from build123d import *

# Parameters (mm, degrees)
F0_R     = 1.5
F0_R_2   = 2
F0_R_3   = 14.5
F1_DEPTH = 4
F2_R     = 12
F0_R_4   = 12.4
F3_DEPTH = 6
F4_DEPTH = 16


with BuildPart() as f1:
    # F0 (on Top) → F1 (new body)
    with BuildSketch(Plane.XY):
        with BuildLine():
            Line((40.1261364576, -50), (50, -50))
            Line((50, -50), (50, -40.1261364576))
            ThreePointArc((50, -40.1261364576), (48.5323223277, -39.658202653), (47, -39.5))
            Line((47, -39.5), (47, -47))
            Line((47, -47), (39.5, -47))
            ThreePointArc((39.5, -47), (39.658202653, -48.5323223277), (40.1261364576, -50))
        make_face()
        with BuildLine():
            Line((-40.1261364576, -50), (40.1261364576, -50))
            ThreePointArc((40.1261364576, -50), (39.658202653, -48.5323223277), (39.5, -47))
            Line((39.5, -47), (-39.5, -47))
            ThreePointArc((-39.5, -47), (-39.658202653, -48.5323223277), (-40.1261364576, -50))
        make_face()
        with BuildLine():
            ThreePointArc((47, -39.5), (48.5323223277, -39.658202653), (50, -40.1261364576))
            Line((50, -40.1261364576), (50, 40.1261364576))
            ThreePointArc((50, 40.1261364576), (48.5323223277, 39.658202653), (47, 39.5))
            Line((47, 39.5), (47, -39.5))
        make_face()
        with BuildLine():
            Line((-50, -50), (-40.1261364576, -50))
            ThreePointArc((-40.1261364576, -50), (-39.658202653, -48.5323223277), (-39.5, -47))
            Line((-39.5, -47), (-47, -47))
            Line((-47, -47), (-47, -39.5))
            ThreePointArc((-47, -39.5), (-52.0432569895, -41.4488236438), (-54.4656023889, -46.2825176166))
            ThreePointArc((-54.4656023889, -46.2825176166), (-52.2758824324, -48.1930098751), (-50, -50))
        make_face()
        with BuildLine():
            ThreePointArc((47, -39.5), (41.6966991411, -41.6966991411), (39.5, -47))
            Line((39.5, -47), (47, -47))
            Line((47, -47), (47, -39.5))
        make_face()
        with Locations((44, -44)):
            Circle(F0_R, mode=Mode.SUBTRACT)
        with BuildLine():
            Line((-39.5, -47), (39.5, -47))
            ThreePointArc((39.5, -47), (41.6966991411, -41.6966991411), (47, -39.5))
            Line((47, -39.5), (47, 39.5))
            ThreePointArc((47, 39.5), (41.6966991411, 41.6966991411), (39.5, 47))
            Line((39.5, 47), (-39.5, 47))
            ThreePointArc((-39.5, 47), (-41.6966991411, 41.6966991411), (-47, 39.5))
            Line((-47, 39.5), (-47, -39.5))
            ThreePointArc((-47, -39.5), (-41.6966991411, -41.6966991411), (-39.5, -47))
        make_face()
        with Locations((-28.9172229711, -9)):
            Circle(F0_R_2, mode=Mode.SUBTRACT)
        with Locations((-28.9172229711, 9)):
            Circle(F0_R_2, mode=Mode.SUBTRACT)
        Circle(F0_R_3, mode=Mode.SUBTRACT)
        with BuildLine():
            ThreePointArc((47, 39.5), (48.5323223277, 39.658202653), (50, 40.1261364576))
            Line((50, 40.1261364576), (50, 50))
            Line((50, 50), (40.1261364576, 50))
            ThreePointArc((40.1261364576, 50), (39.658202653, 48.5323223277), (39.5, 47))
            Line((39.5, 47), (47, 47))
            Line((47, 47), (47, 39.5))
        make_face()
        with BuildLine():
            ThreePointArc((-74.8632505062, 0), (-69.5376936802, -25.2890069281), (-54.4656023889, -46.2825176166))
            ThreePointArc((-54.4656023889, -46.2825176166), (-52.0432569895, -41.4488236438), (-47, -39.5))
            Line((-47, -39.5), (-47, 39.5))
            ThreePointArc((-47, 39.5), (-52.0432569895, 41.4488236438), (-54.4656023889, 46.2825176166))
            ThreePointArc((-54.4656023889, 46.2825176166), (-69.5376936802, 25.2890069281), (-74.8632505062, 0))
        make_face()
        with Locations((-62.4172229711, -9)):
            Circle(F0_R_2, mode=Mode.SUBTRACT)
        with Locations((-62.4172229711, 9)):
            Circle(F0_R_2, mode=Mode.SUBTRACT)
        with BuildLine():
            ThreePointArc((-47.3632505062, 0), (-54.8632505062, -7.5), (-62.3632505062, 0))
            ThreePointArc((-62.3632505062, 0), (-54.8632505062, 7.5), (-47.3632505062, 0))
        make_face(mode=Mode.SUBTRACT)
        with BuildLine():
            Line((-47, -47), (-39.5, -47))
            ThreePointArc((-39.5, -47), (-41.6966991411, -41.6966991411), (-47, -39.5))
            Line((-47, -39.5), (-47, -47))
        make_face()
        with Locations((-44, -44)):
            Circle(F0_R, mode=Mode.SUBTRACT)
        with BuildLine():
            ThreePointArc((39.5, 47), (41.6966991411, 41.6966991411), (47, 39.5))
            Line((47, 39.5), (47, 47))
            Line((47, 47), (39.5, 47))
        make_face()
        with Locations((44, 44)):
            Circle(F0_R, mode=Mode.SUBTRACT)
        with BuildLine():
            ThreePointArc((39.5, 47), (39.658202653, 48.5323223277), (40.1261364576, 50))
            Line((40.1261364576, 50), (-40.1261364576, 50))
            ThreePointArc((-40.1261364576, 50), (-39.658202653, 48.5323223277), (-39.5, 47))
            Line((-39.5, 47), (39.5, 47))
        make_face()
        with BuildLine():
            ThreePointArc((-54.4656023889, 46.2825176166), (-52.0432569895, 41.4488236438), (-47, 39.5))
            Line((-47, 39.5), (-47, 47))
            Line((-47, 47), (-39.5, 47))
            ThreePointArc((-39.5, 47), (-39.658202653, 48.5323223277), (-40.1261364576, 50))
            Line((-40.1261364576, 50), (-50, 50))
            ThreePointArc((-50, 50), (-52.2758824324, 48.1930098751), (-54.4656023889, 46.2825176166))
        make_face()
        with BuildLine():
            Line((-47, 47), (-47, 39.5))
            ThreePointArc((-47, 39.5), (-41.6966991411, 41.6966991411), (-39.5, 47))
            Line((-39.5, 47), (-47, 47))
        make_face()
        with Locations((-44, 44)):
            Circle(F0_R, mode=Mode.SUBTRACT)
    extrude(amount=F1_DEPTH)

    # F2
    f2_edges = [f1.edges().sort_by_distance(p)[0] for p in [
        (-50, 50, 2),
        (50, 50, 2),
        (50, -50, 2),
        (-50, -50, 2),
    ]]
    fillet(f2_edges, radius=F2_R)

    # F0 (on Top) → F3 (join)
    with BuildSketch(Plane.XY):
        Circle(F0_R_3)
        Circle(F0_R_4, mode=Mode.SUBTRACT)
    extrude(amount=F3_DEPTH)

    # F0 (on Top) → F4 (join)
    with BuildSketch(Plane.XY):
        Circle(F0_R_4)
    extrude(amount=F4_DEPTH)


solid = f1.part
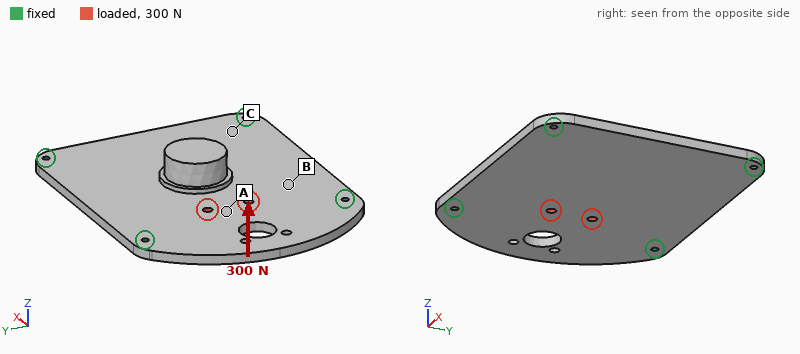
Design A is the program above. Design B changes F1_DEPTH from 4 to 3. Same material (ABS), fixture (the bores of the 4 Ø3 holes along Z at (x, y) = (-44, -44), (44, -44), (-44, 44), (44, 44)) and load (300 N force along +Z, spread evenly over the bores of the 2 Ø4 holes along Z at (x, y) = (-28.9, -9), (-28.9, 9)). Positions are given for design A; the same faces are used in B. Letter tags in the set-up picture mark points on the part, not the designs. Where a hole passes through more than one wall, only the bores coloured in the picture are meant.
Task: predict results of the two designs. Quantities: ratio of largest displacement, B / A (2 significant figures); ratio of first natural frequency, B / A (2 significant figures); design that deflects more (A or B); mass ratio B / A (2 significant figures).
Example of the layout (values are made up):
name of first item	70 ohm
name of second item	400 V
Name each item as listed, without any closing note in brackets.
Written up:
ratio of largest displacement, B / A	2.2
ratio of first natural frequency, B / A	0.73
design that deflects more	B
mass ratio B / A	0.79
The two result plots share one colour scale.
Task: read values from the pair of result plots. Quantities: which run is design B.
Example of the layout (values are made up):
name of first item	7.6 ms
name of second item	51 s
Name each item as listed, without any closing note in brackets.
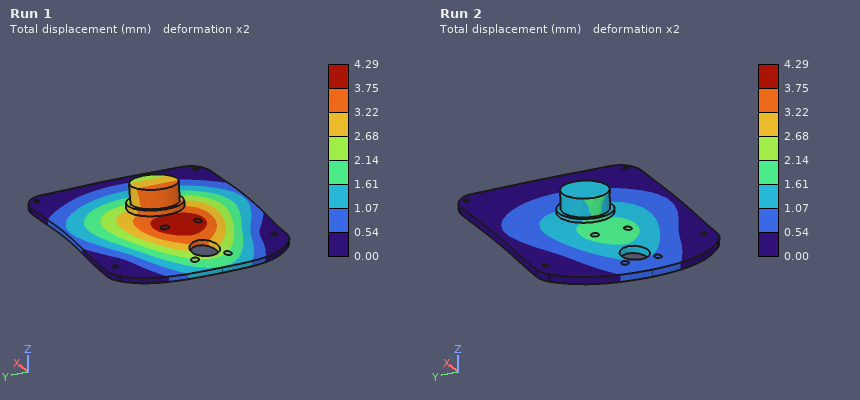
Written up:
which run is design B	Run 1
